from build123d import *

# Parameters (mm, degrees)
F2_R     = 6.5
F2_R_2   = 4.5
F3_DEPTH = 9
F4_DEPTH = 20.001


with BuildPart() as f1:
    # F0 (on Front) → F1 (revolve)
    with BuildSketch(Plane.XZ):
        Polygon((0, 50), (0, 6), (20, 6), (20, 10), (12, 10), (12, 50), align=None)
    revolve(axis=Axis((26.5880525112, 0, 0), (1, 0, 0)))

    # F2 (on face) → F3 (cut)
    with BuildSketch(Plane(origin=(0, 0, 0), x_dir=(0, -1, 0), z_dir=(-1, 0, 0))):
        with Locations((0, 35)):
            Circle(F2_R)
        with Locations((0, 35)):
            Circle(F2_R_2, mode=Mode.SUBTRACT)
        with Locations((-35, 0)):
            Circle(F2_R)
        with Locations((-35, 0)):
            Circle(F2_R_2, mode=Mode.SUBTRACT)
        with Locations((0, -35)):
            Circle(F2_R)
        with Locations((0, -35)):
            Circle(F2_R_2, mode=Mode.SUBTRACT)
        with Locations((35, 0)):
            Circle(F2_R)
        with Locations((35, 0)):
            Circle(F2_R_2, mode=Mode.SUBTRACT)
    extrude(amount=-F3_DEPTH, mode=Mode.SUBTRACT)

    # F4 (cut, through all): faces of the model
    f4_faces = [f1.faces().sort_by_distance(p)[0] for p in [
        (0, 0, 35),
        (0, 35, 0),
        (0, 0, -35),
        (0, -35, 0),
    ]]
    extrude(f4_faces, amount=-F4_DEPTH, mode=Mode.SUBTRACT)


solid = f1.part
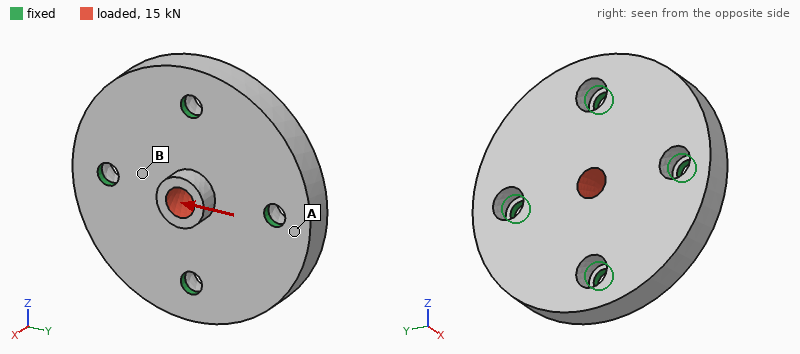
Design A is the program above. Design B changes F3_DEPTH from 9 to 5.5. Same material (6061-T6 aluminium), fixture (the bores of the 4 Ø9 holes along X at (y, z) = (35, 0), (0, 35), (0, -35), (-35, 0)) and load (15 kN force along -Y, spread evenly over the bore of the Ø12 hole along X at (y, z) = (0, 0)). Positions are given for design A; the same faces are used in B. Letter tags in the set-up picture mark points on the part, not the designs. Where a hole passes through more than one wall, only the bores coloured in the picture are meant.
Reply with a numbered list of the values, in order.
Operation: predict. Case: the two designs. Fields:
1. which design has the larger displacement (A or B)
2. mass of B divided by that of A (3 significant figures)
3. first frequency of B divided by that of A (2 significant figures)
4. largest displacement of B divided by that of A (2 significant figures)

1. A
2. 1.01
3. 1.2
4. 0.89
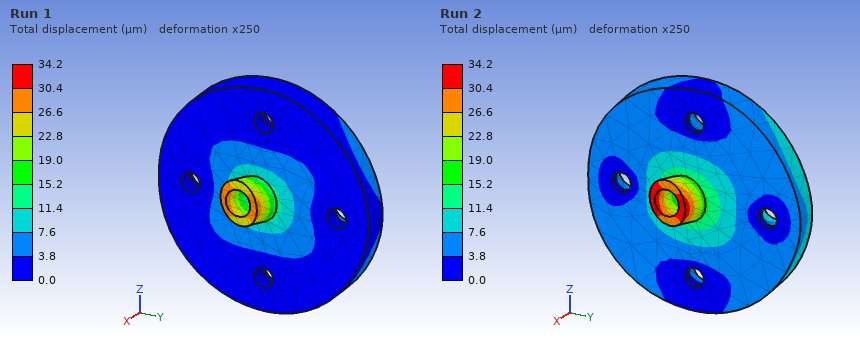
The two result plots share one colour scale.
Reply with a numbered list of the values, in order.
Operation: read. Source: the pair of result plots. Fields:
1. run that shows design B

1. Run 1
